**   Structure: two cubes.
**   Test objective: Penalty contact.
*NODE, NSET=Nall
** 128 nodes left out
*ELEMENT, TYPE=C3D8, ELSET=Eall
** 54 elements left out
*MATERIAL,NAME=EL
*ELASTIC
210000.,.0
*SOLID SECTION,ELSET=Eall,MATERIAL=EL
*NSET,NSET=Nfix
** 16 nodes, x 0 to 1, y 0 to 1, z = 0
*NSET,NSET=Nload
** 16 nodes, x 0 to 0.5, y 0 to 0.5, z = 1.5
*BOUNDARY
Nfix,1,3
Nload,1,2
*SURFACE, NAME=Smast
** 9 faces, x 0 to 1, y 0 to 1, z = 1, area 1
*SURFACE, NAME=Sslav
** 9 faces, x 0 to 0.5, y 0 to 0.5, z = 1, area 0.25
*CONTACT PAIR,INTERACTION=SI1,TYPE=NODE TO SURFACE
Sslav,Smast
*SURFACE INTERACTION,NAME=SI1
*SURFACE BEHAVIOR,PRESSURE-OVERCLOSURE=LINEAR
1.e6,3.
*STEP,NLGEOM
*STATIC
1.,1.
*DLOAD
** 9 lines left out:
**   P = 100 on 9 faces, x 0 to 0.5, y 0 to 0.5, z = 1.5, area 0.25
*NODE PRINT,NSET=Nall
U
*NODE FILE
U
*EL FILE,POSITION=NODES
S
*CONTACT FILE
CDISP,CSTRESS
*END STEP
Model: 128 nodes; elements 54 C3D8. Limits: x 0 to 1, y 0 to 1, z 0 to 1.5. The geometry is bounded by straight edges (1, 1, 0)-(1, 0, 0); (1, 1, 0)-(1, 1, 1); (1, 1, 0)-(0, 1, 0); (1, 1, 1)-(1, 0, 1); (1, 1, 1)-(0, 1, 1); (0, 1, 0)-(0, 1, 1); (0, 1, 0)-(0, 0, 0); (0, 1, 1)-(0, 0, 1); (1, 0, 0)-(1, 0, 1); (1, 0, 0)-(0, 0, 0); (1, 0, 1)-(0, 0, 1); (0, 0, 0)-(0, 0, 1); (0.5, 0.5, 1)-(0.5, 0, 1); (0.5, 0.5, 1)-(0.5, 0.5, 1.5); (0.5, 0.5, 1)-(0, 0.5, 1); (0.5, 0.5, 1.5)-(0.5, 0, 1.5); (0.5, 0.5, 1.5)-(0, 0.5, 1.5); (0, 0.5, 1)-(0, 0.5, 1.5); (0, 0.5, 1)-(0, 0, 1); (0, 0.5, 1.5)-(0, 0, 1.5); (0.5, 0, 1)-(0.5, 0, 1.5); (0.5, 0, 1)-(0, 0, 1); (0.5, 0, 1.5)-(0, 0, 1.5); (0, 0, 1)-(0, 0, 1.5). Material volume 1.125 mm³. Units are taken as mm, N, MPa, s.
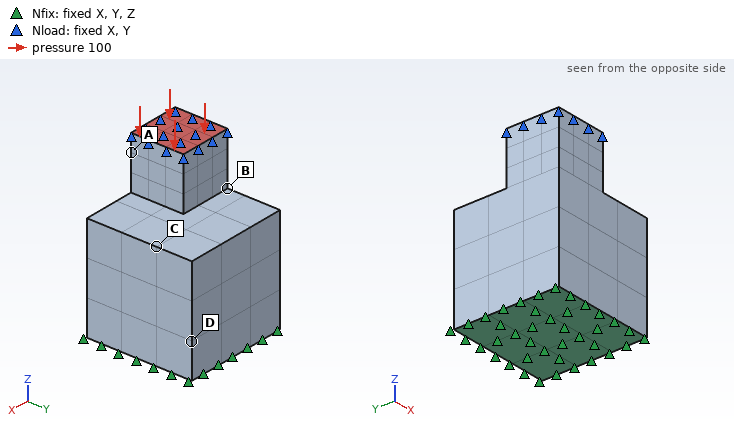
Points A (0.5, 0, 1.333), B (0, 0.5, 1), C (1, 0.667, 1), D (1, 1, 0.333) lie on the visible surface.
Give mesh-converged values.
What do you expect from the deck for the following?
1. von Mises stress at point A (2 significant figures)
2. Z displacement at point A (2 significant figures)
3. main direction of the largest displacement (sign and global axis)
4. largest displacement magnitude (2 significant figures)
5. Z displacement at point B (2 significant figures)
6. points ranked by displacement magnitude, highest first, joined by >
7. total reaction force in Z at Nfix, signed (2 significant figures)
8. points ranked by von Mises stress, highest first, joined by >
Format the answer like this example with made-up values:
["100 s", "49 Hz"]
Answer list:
["100 MPa", "-6.0e-04 mm", "-Z", "9.0e-04 mm", "-4.2e-04 mm", "A > B > C > D", "25 N", "B > A > D > C"]
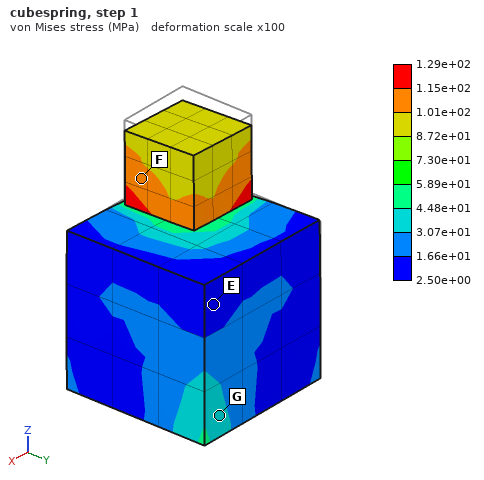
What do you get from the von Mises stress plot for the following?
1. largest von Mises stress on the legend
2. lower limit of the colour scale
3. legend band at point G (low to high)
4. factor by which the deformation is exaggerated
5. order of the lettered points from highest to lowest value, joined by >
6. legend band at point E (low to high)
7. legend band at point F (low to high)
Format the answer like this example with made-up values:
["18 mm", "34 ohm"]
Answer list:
["1.29e+02 MPa", "2.50e+00 MPa", "3.07e+01 to 4.48e+01 MPa", "100", "F > G > E", "2.50e+00 to 1.66e+01 MPa", "1.01e+02 to 1.15e+02 MPa"]
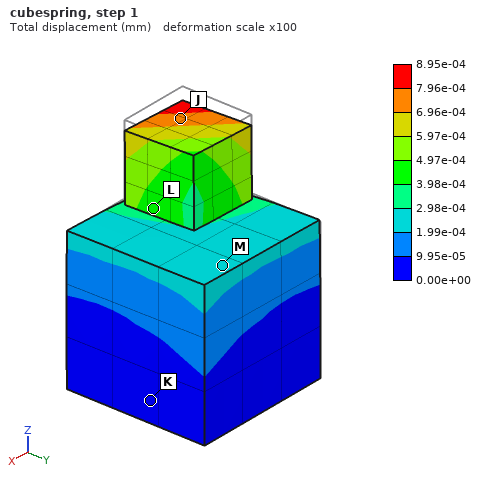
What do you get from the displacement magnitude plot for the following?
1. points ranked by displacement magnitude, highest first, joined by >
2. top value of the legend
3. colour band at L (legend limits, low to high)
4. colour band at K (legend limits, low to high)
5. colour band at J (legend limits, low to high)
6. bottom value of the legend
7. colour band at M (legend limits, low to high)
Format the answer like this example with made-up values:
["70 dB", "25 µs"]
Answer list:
["J > L > M > K", "8.95e-04 mm", "3.98e-04 to 4.97e-04 mm", "0.00e+00 to 9.95e-05 mm", "6.96e-04 to 7.96e-04 mm", "0.00e+00 mm", "1.99e-04 to 2.98e-04 mm"]
